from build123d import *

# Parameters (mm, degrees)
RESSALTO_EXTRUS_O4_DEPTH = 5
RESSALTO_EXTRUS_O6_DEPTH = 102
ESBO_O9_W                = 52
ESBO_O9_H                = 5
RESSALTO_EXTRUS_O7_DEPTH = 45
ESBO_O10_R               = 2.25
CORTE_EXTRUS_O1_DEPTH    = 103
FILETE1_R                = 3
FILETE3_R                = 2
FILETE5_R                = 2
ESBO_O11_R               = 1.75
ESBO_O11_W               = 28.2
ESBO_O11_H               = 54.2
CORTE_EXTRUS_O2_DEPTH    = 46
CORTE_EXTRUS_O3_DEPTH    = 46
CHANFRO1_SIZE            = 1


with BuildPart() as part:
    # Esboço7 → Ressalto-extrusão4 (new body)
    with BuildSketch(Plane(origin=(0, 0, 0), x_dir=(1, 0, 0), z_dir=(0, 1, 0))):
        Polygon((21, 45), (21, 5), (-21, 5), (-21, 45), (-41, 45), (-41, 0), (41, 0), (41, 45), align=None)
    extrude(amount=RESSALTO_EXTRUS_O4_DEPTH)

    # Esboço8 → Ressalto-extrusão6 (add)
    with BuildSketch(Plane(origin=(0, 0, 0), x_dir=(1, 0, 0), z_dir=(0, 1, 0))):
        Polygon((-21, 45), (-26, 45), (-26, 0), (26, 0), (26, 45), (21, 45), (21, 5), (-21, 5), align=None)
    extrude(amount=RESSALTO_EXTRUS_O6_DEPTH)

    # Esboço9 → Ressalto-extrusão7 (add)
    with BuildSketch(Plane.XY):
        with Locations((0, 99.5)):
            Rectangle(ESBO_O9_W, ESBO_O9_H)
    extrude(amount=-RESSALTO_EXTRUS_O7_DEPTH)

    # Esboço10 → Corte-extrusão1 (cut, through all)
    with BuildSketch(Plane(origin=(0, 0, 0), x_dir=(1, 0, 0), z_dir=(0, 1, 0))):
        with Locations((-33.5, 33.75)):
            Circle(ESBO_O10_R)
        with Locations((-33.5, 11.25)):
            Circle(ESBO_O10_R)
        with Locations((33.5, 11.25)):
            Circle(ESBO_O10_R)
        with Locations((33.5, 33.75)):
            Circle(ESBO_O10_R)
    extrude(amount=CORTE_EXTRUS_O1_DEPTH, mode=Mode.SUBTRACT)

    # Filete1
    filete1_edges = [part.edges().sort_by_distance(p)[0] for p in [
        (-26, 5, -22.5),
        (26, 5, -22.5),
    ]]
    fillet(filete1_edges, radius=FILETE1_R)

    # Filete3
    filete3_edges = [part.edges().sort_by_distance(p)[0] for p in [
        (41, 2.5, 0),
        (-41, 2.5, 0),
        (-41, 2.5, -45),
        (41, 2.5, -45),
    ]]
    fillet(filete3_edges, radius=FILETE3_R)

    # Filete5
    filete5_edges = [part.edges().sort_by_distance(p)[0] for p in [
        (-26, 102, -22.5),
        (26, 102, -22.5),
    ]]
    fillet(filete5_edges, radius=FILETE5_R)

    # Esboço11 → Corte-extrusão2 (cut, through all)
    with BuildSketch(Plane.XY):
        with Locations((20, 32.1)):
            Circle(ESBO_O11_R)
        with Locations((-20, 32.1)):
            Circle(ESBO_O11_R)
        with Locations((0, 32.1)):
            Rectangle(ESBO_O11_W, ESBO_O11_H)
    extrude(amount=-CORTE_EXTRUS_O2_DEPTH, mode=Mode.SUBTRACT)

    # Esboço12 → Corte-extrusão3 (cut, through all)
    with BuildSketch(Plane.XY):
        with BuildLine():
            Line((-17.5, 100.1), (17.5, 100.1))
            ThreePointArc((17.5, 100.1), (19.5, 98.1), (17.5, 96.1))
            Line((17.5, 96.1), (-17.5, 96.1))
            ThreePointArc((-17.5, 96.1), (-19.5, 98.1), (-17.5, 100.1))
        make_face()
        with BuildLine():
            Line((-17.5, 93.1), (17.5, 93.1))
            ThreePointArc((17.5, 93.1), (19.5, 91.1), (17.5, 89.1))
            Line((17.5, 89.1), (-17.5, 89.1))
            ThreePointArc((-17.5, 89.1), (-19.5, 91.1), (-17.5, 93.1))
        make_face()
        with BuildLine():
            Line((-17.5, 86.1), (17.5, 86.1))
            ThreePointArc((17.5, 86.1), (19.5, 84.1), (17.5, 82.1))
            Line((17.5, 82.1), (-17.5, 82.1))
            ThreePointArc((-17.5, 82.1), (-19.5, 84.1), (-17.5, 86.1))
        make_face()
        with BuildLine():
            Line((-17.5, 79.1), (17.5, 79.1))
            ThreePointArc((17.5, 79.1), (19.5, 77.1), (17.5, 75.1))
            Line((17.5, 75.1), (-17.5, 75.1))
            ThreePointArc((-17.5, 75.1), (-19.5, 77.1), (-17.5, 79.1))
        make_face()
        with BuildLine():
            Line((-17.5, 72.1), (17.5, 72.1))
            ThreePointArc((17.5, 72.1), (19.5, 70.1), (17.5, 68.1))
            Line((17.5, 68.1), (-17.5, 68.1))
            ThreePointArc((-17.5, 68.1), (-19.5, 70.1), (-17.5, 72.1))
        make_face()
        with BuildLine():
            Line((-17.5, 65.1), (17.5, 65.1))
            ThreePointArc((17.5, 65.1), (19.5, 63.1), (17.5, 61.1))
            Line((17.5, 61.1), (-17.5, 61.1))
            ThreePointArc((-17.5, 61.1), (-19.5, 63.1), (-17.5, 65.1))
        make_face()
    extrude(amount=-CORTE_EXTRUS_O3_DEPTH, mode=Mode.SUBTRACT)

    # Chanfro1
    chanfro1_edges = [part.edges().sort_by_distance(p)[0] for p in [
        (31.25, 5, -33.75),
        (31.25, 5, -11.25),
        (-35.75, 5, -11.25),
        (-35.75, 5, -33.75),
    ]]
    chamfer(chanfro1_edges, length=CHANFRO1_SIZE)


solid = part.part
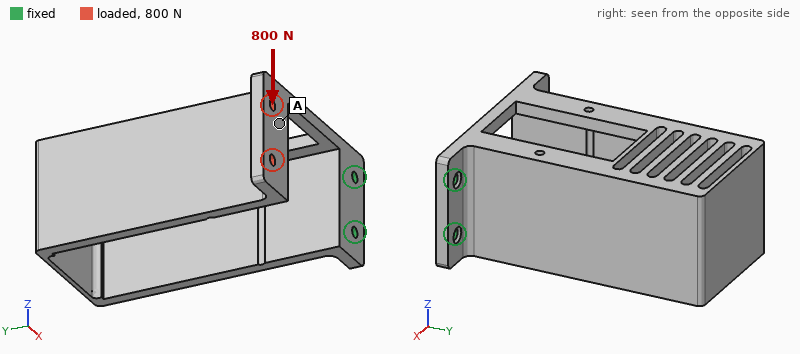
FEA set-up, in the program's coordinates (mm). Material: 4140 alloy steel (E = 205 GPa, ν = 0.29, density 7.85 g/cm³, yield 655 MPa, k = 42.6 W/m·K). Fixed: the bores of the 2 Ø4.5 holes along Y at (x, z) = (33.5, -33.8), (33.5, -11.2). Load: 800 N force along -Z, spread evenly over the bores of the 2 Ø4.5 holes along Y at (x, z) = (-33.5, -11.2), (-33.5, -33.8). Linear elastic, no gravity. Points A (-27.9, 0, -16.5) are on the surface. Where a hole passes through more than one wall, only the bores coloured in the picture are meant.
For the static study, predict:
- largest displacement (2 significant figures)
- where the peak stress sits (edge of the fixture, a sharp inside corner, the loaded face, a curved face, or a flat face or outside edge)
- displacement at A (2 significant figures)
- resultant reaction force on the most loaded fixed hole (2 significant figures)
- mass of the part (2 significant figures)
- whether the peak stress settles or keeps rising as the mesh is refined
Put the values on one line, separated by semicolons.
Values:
1.6 mm; a sharp inside corner; 1.1 mm; 2.2 kN; 510 g; keeps rising
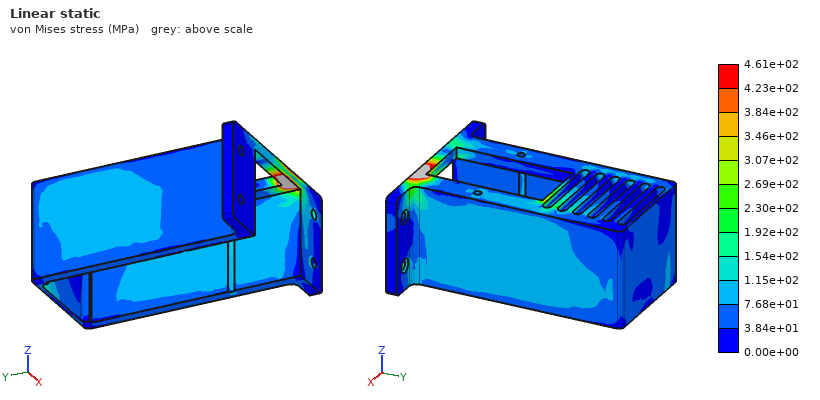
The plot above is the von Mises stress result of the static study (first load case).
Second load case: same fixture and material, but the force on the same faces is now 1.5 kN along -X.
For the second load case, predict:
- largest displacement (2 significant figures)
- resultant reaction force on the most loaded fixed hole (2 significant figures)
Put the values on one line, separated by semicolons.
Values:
1.5 mm; 790 N
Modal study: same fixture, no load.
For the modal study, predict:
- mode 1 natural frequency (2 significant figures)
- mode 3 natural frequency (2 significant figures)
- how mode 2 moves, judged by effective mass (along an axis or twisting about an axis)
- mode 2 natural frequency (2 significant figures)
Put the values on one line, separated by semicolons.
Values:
230 Hz; 700 Hz; along Z; 330 Hz
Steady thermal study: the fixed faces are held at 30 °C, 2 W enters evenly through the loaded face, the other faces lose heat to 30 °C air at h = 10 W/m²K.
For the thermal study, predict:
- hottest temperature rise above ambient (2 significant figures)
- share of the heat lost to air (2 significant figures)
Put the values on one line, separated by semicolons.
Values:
15 K; 78 %
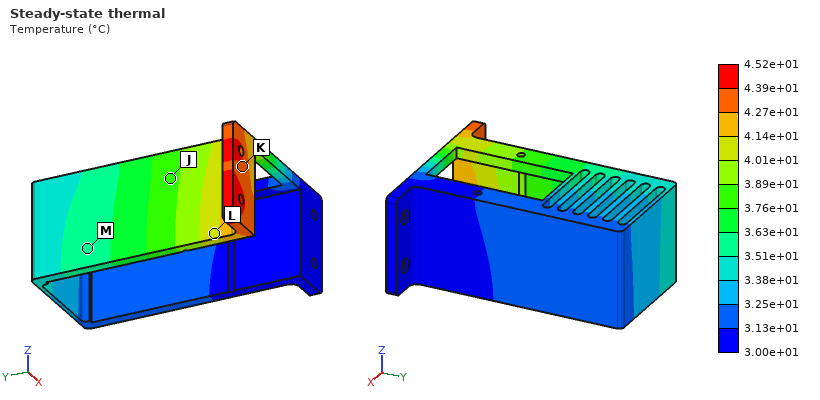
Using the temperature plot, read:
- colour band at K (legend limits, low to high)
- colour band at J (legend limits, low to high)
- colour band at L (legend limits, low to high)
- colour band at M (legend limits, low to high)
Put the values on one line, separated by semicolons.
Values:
4.27e+01 to 4.39e+01 °C; 3.76e+01 to 3.89e+01 °C; 4.01e+01 to 4.14e+01 °C; 3.51e+01 to 3.63e+01 °C
